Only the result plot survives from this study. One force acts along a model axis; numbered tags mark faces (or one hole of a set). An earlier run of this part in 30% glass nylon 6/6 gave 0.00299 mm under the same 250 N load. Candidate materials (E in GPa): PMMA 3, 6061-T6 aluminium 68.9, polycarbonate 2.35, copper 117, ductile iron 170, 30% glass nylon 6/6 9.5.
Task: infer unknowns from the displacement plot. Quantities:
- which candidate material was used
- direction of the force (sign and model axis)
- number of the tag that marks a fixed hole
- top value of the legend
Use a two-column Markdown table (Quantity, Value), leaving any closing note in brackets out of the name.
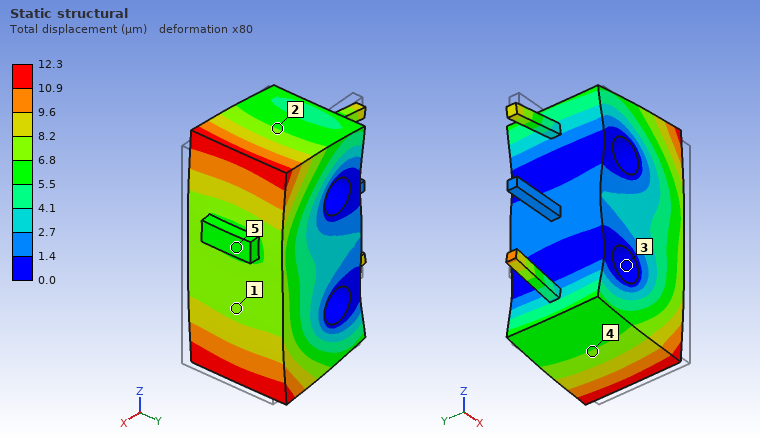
| Quantity | Value |
|---|---|
| which candidate material was used | polycarbonate |
| direction of the force | -X |
| number of the tag that marks a fixed hole | 3 |
| top value of the legend | 12.3 µm |
